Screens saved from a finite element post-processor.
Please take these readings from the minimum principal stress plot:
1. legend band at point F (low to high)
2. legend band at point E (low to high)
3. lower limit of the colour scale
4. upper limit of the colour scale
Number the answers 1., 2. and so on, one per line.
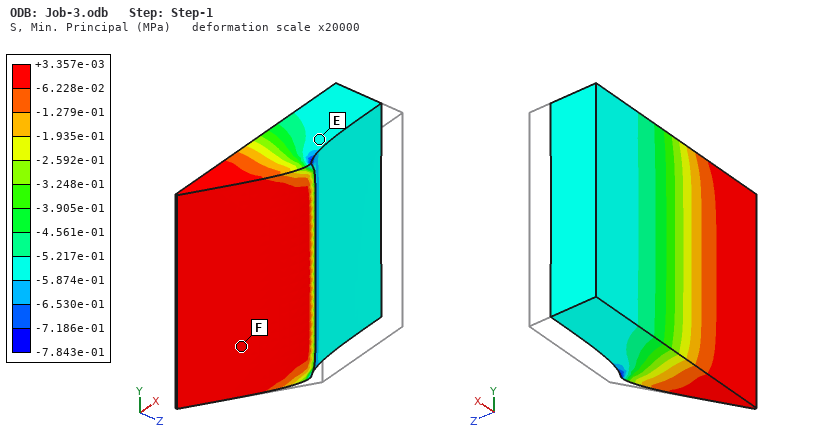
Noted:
1. -6.228e-02 to +3.357e-03 MPa
2. -5.874e-01 to -5.217e-01 MPa
3. -7.843e-01 MPa
4. +3.357e-03 MPa
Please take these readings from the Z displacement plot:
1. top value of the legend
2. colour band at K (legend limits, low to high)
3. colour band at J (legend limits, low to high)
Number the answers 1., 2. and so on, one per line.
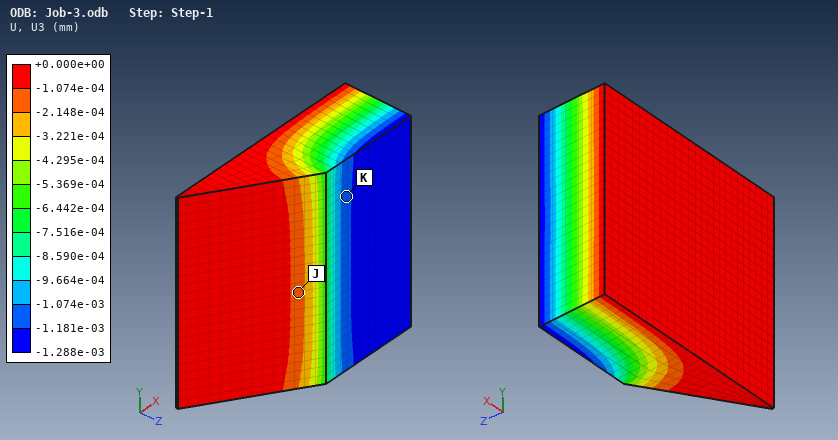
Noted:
1. +0.000e+00 mm
2. -1.181e-03 to -1.074e-03 mm
3. -2.148e-04 to -1.074e-04 mm
